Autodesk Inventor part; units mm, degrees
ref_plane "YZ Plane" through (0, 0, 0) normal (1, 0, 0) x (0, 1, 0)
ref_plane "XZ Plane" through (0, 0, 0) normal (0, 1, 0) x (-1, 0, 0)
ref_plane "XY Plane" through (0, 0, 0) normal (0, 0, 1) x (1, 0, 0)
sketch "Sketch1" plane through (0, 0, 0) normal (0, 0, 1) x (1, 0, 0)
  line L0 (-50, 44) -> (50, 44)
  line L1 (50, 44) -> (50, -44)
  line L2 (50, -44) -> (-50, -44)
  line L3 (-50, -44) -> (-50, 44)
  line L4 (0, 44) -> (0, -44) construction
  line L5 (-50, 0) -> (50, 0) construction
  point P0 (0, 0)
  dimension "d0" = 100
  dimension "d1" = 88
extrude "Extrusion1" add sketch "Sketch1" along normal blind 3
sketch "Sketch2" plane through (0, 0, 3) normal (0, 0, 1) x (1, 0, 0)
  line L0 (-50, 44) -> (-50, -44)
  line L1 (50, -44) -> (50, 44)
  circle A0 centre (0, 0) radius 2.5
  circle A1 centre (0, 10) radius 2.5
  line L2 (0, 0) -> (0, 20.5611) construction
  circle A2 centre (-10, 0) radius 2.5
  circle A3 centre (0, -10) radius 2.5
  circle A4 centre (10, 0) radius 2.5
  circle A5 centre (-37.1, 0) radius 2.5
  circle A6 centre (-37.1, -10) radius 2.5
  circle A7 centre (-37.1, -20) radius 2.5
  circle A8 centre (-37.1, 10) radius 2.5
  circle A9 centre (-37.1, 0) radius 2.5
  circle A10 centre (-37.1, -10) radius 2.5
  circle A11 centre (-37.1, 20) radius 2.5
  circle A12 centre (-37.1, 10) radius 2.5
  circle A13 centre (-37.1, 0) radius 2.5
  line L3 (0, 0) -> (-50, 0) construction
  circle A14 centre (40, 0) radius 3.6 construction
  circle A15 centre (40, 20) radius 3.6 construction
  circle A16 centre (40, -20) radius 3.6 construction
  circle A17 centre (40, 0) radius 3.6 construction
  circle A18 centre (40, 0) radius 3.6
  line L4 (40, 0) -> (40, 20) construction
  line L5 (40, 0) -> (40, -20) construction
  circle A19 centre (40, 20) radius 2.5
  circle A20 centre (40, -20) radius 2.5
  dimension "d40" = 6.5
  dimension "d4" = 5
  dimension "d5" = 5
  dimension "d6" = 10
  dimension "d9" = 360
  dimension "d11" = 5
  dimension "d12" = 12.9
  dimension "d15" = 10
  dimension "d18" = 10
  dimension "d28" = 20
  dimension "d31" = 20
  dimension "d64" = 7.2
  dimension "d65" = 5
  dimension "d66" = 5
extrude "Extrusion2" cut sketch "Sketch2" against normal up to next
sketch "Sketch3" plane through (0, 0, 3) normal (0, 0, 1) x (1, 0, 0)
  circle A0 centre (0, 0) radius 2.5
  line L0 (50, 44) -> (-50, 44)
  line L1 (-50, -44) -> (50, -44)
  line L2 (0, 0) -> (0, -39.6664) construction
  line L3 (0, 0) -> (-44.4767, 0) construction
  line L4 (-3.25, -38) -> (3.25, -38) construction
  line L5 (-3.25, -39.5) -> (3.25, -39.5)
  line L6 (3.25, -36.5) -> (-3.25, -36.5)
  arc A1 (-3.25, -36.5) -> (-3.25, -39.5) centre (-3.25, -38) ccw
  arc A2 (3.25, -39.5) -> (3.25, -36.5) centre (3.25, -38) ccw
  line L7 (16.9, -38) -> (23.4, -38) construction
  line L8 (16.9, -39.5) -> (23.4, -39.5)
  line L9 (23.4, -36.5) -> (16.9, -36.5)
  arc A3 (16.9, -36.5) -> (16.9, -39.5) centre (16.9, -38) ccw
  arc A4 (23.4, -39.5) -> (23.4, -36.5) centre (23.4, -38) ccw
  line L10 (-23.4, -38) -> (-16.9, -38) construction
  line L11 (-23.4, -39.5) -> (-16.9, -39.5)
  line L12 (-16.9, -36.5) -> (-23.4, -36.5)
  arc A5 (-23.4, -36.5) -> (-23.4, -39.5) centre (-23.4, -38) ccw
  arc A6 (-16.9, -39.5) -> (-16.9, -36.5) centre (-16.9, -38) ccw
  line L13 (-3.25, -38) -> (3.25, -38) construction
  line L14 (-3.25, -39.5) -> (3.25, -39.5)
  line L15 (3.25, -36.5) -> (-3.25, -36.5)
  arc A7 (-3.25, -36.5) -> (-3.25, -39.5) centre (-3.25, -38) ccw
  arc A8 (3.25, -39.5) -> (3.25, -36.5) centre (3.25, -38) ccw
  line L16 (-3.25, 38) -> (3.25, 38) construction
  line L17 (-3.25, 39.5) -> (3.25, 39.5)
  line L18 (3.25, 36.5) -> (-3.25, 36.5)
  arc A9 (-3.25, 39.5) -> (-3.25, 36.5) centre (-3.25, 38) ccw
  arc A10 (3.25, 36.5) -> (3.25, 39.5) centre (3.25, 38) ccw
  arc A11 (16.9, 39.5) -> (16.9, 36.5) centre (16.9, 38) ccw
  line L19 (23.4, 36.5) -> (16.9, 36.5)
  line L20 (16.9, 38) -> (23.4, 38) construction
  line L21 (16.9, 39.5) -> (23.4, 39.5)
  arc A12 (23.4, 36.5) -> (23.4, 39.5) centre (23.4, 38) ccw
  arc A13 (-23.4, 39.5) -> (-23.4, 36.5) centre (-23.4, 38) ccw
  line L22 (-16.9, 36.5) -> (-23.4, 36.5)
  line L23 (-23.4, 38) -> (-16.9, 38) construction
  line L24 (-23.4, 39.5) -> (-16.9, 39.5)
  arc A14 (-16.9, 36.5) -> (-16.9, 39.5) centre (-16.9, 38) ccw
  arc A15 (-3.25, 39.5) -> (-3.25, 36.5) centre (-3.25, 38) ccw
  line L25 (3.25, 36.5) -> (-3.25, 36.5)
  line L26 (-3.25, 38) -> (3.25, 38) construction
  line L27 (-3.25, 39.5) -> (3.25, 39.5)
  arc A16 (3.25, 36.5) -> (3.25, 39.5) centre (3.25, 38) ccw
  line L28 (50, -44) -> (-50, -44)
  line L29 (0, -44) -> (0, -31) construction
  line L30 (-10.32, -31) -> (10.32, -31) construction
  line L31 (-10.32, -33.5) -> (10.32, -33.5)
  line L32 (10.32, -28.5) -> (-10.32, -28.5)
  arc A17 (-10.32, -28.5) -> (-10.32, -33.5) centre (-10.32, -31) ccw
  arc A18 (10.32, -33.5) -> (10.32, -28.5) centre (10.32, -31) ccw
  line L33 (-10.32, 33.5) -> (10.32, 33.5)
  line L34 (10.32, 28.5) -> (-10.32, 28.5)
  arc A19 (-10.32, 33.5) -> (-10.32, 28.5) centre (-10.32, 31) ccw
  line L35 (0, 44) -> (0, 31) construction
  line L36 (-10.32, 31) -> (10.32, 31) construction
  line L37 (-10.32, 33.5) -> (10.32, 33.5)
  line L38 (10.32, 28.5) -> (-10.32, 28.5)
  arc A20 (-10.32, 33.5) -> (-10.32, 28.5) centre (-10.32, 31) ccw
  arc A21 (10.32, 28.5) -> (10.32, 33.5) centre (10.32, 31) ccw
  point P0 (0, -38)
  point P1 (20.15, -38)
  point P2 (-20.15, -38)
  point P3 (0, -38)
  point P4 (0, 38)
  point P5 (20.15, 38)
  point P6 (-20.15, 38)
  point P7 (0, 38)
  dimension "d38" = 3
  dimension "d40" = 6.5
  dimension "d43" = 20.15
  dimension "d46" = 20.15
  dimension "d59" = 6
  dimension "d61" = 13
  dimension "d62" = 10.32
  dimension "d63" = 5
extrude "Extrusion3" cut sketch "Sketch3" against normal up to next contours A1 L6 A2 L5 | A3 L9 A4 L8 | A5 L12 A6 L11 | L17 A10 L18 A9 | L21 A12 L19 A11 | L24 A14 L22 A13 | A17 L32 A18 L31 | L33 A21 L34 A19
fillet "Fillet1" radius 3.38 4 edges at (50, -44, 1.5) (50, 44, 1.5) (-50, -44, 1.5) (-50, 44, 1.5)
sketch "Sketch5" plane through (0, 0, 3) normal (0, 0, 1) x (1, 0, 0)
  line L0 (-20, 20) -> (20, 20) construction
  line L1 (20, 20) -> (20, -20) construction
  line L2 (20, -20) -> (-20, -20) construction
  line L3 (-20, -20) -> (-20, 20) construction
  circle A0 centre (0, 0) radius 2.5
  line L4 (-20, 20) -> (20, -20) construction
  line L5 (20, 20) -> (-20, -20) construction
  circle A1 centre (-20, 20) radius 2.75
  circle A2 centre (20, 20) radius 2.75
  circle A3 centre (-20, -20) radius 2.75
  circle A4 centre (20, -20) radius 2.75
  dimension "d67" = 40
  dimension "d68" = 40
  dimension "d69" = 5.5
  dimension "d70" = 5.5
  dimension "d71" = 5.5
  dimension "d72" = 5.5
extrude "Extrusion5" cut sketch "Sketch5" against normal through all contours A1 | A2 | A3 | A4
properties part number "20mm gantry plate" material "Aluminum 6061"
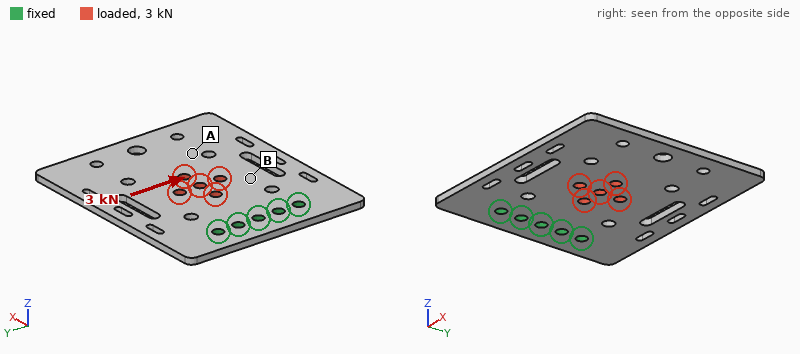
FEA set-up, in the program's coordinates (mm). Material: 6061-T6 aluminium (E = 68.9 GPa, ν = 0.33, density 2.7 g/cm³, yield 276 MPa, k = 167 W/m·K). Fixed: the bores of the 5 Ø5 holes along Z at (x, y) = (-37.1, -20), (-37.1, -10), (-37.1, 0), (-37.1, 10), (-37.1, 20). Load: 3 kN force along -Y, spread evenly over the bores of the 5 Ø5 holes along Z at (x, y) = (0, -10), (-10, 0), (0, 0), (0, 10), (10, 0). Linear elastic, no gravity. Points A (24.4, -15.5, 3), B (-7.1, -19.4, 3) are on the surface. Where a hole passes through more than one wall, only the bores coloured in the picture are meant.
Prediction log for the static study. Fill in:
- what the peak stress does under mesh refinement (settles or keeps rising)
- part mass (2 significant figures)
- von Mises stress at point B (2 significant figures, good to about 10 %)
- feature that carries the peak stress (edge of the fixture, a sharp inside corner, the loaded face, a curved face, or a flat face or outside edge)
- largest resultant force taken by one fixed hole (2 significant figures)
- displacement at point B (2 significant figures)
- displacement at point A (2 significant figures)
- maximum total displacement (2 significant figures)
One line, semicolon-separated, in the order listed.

keeps rising; 65 g; 25 MPa; edge of the fixture; 2.4 kN; 36 µm; 63 µm; 83 µm
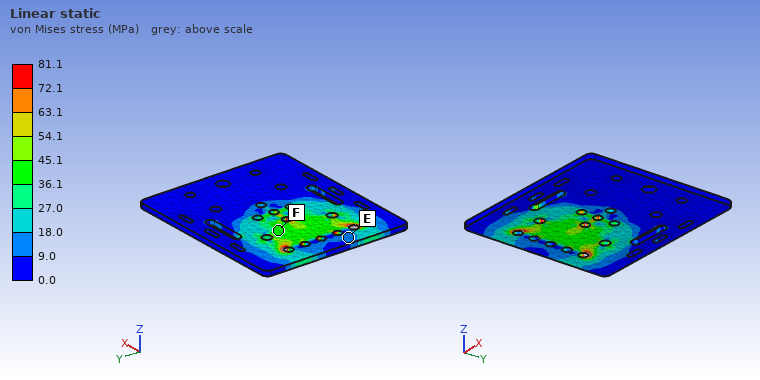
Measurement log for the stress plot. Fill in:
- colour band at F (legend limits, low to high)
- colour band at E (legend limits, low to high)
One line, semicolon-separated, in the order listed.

36.1 to 45.1 MPa; 9.0 to 18.0 MPa
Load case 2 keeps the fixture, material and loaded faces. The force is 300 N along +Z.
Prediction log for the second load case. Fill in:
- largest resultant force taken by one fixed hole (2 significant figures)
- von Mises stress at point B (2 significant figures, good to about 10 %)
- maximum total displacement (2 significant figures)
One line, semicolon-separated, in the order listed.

77 N; 22 MPa; 1.2 mm
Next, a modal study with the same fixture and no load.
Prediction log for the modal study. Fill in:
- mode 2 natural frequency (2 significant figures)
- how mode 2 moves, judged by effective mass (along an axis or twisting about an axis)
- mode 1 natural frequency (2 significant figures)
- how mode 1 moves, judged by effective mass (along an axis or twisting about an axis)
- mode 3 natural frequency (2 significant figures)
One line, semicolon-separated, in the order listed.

710 Hz; twisting about X; 320 Hz; along Z; 1900 Hz
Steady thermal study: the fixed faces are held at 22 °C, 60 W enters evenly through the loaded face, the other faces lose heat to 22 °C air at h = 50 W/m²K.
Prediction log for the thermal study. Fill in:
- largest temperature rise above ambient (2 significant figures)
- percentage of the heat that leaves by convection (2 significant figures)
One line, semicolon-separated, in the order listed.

56 K; 36 %
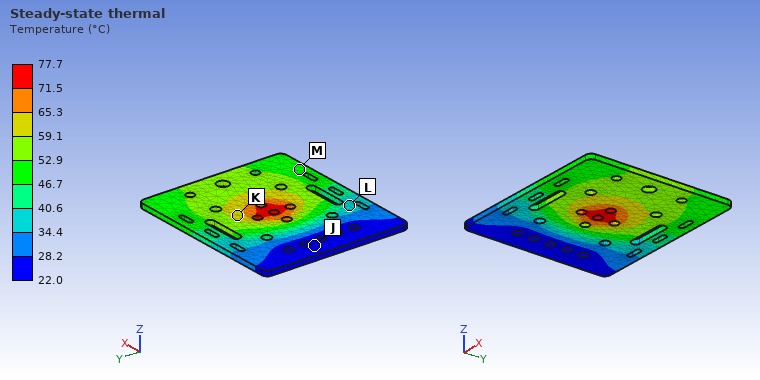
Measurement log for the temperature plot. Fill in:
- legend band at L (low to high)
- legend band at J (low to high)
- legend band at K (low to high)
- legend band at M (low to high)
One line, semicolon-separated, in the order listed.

34.4 to 40.6 °C; 22.0 to 28.2 °C; 59.1 to 65.3 °C; 46.7 to 52.9 °C
